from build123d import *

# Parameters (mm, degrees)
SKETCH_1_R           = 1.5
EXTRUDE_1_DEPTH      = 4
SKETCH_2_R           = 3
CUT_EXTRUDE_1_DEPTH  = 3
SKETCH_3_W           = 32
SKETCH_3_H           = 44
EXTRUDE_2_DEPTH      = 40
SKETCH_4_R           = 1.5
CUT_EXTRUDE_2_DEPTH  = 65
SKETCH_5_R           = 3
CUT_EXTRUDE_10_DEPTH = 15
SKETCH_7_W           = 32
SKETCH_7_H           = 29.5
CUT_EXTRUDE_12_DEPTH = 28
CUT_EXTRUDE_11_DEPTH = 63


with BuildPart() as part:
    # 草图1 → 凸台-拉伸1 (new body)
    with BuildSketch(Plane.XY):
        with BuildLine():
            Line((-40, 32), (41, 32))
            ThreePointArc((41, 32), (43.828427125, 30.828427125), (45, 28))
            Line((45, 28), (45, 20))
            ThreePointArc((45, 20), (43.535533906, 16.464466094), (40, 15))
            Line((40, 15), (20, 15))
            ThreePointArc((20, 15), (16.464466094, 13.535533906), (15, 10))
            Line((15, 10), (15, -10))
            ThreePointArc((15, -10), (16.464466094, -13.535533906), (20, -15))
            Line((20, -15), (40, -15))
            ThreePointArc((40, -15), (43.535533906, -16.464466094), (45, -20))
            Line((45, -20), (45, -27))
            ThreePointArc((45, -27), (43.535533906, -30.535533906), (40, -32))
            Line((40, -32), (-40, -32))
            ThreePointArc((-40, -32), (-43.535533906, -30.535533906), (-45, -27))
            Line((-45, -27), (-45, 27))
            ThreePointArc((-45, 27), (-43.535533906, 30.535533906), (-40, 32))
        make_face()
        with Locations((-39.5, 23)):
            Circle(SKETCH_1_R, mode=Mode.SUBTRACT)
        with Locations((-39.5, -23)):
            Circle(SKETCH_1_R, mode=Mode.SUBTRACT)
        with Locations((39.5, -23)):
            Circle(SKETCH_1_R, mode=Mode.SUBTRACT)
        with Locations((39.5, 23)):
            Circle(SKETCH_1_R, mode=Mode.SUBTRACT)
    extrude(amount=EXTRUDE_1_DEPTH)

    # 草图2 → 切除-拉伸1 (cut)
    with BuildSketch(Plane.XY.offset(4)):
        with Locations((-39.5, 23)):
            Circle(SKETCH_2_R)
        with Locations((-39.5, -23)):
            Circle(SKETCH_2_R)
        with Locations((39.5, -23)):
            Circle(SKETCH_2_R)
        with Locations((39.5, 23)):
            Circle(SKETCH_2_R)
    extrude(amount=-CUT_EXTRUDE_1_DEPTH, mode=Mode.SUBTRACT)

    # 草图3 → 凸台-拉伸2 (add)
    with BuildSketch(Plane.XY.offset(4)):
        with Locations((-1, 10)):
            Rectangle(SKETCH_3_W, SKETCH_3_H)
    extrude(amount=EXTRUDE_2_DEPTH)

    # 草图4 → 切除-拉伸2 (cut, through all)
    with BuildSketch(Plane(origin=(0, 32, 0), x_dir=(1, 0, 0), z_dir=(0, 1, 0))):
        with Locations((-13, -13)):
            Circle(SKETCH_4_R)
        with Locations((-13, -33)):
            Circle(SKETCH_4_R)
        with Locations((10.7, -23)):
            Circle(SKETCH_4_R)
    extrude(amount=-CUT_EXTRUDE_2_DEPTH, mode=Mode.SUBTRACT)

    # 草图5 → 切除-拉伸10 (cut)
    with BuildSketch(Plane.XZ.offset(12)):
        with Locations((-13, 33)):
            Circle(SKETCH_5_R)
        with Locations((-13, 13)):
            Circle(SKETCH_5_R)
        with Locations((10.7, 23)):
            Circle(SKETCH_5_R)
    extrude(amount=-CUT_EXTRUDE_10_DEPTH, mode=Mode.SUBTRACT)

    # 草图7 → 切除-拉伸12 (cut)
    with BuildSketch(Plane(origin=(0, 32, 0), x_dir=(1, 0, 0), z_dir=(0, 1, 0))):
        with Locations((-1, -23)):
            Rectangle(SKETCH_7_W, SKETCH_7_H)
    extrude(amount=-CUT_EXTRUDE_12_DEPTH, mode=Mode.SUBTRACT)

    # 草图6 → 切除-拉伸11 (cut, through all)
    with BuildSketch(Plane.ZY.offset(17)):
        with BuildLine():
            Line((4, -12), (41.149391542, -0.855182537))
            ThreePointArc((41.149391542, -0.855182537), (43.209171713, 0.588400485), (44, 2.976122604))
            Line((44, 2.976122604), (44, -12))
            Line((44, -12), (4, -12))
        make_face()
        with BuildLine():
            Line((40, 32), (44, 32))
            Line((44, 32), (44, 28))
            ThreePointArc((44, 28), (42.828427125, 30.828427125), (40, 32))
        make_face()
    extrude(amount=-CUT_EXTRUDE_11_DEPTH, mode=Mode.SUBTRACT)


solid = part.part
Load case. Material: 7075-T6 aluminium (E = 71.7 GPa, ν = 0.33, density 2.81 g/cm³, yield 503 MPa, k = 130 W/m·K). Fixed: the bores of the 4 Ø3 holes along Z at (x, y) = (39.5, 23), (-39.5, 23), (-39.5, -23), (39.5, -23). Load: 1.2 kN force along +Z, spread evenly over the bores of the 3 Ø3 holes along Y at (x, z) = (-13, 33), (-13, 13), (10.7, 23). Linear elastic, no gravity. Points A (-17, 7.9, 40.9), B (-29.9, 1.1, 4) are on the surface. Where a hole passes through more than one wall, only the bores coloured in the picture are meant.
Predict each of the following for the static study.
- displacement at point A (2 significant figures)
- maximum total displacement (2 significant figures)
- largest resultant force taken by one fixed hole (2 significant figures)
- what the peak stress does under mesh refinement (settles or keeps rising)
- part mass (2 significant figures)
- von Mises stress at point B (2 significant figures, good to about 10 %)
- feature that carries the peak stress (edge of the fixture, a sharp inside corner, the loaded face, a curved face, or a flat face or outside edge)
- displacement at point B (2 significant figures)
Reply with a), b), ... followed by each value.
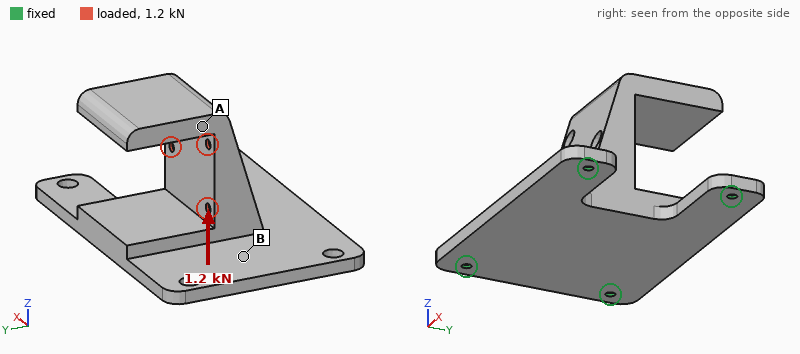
a) 0.14 mm
b) 0.17 mm
c) 1.1 kN
d) keeps rising
e) 110 g
f) 24 MPa
g) edge of the fixture
h) 0.077 mm
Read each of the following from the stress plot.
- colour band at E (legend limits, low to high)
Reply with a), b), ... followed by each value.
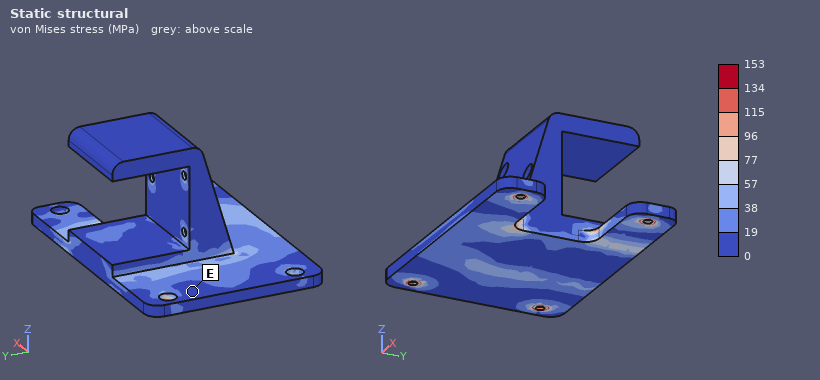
a) 0 to 19 MPa
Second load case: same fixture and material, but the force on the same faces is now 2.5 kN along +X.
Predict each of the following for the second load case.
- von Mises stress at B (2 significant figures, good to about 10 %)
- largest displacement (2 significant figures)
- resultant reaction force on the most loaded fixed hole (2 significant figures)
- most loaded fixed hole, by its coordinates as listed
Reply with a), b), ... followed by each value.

a) 39 MPa
b) 0.35 mm
c) 1.1 kN
d) (39.5, 23)
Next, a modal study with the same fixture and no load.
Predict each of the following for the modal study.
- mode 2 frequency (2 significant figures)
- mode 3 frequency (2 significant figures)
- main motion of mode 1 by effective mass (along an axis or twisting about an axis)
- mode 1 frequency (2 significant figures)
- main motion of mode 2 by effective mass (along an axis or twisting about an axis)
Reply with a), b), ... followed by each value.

a) 1400 Hz
b) 2100 Hz
c) along Y
d) 1400 Hz
e) along Z
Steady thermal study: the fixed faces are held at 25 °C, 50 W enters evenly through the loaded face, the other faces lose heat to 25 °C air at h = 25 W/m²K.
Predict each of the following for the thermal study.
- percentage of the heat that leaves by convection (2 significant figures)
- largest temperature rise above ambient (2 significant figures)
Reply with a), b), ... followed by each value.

a) 29 %
b) 83 K
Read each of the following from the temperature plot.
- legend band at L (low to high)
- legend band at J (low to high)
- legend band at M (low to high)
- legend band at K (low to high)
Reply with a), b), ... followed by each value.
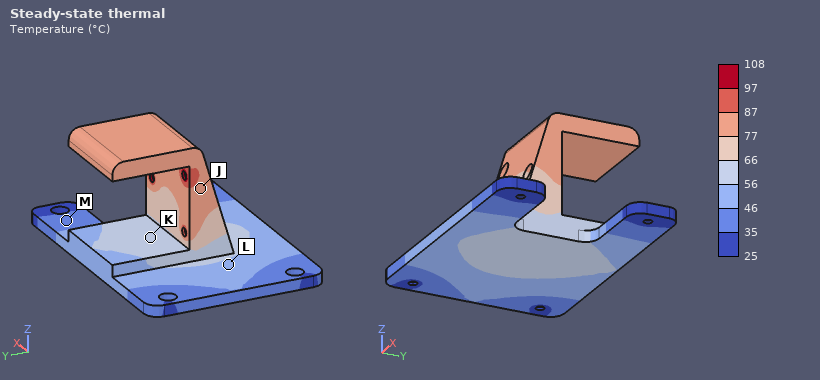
a) 46 to 56 °C
b) 77 to 87 °C
c) 35 to 46 °C
d) 56 to 66 °C
